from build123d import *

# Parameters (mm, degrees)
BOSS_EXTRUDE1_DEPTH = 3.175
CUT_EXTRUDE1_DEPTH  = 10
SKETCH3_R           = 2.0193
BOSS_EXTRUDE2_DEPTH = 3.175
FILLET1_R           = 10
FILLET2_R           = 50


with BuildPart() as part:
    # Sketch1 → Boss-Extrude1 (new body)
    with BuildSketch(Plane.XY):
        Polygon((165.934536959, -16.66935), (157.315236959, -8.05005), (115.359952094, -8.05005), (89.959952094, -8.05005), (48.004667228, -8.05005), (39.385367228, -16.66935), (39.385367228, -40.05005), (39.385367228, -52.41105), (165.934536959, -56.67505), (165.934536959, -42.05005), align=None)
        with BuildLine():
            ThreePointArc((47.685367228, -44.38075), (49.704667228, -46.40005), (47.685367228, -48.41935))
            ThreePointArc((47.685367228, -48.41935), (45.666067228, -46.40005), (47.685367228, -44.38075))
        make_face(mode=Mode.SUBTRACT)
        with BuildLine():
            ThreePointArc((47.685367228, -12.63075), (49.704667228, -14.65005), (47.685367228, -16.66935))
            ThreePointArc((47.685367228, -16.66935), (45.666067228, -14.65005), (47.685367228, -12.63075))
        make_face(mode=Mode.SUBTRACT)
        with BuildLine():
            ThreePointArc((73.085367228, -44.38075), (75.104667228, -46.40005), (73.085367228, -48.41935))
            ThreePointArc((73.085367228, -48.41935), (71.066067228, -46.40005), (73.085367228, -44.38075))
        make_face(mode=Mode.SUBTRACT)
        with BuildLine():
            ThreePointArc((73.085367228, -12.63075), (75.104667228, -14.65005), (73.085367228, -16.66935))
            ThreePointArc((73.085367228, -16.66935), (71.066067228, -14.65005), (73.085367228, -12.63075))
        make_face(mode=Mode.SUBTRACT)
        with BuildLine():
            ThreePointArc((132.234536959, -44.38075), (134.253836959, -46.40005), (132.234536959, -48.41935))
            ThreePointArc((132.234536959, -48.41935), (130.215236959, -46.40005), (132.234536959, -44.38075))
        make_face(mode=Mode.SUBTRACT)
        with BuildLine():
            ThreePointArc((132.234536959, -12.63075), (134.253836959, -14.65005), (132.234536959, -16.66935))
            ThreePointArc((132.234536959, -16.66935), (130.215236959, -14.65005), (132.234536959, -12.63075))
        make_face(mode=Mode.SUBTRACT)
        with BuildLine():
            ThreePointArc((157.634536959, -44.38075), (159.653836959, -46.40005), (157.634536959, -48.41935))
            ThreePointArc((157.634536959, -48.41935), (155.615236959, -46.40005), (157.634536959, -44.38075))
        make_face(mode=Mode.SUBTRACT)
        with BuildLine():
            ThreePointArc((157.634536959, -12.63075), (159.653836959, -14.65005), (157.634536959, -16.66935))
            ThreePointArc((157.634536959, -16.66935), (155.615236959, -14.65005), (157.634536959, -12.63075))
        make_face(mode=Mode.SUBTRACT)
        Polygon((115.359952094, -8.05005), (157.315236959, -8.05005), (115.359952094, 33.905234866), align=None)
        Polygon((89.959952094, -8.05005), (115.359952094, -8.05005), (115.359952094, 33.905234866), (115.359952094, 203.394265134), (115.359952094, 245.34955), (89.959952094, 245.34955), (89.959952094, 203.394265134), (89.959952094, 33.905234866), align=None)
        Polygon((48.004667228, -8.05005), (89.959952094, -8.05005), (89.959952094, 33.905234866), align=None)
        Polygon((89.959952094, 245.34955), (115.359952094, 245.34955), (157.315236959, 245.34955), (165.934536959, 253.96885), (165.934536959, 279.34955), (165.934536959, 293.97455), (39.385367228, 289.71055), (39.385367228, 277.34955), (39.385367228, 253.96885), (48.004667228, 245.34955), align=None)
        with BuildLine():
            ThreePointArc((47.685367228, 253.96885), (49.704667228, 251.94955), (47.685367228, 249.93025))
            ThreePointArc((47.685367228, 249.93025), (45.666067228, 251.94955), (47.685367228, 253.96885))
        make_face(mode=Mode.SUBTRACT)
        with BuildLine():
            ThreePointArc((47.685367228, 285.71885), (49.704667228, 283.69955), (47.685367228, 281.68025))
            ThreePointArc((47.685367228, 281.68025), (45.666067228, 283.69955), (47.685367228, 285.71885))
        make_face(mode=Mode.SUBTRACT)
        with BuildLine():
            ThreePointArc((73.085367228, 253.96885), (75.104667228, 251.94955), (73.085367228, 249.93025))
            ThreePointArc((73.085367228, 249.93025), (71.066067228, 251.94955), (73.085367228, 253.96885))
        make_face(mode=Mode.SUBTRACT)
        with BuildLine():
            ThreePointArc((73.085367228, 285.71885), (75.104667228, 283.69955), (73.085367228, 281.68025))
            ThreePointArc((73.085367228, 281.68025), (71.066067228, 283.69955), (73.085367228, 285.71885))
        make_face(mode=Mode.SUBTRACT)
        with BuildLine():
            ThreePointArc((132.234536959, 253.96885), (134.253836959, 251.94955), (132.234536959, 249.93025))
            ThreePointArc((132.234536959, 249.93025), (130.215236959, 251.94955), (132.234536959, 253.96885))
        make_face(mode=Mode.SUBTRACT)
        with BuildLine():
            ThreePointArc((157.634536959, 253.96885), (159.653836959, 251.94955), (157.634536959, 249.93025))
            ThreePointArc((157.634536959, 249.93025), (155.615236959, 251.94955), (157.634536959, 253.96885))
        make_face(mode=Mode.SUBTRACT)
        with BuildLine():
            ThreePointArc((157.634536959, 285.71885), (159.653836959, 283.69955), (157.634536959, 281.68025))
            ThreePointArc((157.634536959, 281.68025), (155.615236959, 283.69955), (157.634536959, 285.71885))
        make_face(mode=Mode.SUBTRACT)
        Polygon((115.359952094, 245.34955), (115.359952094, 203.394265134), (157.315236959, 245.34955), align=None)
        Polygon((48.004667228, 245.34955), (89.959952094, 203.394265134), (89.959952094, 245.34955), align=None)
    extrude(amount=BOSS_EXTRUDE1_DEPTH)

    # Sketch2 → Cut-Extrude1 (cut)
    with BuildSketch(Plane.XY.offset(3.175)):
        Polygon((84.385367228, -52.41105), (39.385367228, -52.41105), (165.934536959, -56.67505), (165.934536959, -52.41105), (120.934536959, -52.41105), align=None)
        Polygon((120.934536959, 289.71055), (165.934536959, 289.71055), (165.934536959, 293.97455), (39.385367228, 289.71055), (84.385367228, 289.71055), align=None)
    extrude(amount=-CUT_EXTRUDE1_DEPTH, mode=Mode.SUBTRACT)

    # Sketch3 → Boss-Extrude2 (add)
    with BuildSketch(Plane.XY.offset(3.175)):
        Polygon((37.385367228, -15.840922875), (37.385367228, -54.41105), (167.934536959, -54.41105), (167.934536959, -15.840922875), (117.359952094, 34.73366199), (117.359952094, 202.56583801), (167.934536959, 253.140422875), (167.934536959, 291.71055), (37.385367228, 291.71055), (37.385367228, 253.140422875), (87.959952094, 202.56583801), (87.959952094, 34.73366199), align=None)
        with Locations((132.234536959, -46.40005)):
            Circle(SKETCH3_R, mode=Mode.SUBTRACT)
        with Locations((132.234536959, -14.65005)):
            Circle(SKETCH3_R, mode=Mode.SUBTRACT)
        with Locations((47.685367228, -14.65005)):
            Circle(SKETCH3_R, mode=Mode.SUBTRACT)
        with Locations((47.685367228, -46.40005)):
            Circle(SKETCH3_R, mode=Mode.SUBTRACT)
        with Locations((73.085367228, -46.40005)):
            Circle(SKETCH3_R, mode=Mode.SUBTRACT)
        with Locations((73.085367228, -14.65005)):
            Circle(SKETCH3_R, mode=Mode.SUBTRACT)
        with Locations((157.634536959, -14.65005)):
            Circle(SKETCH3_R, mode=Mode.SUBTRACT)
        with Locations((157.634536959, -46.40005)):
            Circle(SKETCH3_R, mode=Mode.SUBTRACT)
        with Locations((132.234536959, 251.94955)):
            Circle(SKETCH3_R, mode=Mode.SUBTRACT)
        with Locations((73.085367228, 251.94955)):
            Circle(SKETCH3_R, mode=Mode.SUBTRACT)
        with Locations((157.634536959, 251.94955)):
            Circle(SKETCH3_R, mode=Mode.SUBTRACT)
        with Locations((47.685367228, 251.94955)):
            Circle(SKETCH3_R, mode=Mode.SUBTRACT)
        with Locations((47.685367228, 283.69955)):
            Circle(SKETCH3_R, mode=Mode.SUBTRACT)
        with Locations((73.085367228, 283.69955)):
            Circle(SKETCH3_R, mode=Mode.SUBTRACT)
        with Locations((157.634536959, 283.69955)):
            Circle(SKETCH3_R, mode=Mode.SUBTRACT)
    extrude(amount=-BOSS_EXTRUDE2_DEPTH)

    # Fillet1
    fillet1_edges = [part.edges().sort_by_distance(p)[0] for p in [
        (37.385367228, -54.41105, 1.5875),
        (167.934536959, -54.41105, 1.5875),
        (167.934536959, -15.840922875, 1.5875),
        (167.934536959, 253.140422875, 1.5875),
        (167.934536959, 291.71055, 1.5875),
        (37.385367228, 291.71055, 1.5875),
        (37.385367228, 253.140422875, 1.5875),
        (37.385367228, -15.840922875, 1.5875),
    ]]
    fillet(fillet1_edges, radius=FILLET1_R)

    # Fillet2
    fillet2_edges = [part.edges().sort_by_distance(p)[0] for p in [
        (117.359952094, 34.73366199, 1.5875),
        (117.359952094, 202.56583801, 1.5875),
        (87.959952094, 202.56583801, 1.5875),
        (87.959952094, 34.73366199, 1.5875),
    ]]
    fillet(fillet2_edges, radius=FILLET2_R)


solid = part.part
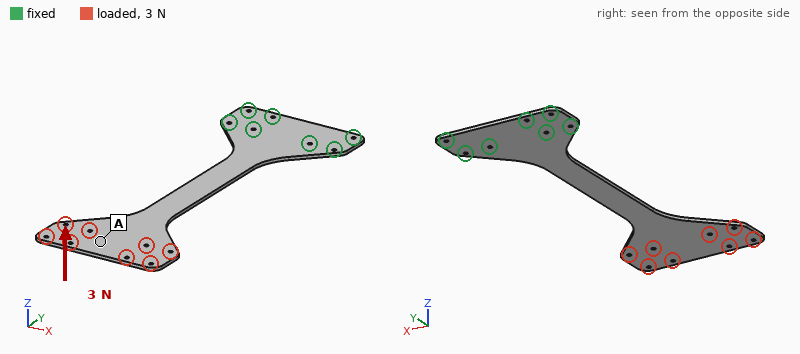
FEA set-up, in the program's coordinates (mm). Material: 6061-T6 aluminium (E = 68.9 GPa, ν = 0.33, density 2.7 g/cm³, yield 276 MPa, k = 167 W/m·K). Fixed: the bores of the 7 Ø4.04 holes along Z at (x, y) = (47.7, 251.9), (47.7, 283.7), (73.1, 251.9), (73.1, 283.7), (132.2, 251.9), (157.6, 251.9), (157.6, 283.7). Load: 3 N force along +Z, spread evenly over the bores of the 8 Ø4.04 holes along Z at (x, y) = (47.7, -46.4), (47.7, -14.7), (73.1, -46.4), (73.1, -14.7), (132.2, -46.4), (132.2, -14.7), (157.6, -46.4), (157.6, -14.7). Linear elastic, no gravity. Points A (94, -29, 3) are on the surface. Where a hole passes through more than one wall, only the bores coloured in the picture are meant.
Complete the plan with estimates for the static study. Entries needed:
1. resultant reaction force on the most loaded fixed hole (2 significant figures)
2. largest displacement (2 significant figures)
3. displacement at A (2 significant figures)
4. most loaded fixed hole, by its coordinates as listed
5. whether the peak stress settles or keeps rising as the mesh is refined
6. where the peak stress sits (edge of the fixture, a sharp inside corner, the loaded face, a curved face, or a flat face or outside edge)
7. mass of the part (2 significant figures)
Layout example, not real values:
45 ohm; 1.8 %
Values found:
10 N; 3.6 mm; 3.1 mm; (73.1, 251.9); keeps rising; edge of the fixture; 200 g
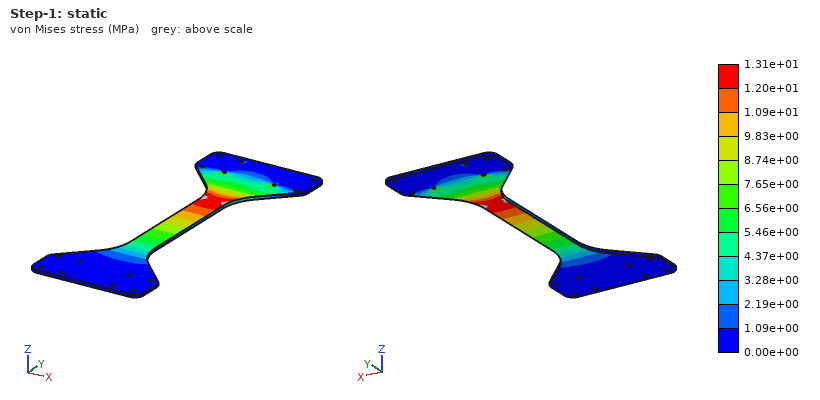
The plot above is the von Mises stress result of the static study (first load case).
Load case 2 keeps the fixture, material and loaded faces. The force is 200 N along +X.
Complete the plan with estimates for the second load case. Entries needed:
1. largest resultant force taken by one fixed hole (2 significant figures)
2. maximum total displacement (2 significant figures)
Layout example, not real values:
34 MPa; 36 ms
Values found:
510 N; 2.3 mm
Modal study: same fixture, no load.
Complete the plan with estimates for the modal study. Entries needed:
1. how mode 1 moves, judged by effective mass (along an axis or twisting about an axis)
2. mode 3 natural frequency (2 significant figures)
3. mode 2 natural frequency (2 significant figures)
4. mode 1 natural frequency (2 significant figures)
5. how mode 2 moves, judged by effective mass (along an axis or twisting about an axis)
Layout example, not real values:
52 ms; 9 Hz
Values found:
along Z; 170 Hz; 110 Hz; 18 Hz; twisting about Y
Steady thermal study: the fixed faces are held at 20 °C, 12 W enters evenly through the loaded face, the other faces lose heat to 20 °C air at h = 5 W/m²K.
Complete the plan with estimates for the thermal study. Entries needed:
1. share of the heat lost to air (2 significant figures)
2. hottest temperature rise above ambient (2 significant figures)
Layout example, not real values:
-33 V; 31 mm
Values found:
67 %; 70 K
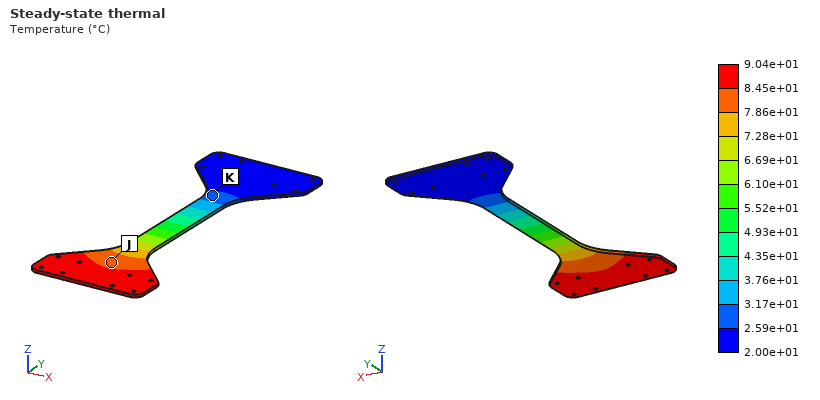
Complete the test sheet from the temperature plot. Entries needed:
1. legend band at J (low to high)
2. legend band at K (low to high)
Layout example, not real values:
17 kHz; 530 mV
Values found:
7.86e+01 to 8.45e+01 °C; 2.59e+01 to 3.17e+01 °C
